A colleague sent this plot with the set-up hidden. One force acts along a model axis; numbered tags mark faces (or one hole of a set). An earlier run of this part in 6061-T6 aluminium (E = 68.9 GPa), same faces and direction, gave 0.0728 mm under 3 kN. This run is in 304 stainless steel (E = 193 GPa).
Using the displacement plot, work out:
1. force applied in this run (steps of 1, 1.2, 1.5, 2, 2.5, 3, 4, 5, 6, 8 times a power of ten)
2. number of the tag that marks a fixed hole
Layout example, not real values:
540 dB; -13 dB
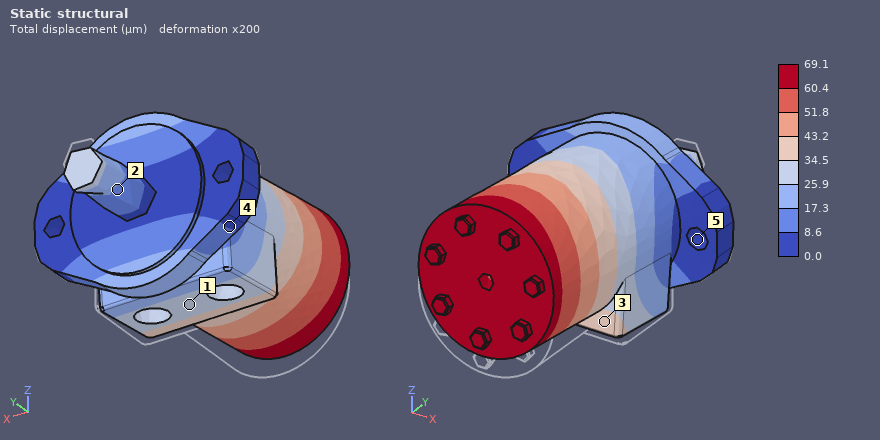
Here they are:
8 kN; 5
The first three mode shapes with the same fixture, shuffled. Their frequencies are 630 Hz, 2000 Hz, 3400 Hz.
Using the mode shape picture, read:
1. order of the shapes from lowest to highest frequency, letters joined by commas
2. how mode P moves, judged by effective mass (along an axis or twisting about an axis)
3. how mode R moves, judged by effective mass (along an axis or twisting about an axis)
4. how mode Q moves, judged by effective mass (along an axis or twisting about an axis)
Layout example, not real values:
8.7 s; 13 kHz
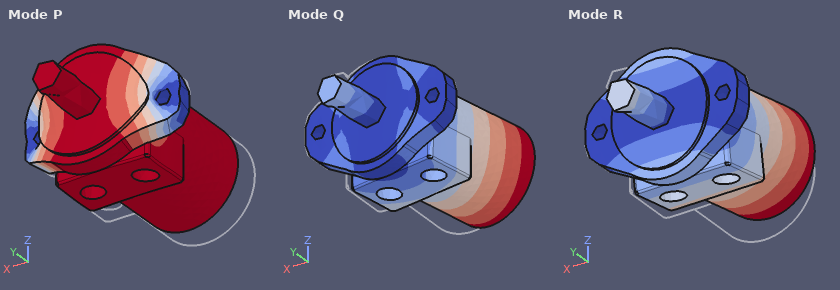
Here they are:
R, Q, P; along Y; along Z; along X
